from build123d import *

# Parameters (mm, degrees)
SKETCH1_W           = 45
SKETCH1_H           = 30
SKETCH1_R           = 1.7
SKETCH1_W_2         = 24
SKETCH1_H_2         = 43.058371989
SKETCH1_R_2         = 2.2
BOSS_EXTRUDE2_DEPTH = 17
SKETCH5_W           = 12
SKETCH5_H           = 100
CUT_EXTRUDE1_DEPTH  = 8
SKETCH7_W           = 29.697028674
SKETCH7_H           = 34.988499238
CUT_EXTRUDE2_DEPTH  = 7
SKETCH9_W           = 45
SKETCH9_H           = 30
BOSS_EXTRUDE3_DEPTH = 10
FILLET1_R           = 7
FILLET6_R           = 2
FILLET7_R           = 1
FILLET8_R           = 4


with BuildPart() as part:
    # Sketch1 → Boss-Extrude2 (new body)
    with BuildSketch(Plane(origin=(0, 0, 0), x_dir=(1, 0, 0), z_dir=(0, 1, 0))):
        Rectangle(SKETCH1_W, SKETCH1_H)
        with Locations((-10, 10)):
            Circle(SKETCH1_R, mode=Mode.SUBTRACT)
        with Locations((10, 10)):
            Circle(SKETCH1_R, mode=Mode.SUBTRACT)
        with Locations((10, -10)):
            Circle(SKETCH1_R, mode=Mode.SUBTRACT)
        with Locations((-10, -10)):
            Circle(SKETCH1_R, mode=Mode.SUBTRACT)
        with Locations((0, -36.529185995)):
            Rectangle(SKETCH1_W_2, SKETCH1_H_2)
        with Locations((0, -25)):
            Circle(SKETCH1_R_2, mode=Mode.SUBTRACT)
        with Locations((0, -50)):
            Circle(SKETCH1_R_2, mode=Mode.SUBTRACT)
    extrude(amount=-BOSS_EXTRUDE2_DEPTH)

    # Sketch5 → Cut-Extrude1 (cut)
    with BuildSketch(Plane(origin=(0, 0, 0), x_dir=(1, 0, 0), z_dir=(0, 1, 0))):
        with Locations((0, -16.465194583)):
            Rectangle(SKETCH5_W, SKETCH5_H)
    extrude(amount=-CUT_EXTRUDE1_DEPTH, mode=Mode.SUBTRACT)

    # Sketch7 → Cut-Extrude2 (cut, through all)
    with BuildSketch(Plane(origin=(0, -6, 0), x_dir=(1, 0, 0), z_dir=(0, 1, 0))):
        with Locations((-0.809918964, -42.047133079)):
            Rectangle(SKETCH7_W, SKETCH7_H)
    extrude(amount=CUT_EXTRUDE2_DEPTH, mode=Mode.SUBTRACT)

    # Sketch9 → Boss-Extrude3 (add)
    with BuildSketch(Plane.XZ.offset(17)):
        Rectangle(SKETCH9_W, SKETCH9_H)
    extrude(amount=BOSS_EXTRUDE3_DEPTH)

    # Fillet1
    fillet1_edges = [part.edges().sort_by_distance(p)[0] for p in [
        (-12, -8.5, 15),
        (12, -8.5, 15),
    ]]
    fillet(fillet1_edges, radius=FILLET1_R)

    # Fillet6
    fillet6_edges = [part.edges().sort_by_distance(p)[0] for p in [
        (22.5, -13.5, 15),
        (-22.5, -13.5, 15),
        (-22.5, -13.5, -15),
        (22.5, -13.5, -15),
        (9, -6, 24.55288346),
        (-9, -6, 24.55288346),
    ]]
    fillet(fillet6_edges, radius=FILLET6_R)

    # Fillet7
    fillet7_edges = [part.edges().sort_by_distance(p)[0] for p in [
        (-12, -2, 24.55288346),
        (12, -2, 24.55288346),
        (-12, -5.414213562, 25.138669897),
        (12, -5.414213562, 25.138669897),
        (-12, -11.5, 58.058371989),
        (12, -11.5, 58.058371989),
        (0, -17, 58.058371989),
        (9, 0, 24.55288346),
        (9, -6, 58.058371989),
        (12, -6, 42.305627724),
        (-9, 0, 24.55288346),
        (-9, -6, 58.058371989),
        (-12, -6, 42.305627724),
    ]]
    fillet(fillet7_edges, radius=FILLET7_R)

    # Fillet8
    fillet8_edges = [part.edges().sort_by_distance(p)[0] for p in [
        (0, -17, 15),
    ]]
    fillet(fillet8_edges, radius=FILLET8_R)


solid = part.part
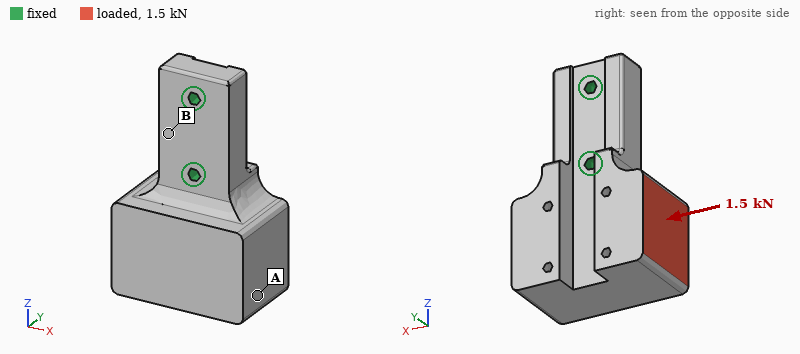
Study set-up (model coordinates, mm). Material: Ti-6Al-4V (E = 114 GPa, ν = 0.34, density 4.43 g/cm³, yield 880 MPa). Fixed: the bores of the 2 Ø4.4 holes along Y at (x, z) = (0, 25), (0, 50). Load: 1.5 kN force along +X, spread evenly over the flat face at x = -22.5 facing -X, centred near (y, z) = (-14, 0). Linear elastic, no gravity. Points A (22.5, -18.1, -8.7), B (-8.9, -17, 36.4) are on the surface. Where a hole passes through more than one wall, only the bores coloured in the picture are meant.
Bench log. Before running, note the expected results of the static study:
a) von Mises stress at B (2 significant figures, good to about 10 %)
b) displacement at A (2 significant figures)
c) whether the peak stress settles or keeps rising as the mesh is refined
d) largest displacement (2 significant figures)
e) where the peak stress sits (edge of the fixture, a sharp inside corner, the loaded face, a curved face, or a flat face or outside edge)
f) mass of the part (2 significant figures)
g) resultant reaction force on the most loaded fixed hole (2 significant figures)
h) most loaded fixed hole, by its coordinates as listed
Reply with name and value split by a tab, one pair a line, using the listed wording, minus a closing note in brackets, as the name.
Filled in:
von Mises stress at B	13 MPa
displacement at A	25 µm
whether the peak stress settles or keeps rising as the mesh is refined	keeps rising
largest displacement	28 µm
where the peak stress sits	edge of the fixture
mass of the part	200 g
resultant reaction force on the most loaded fixed hole	2.6 kN
most loaded fixed hole, by its coordinates as listed	(0, 25)
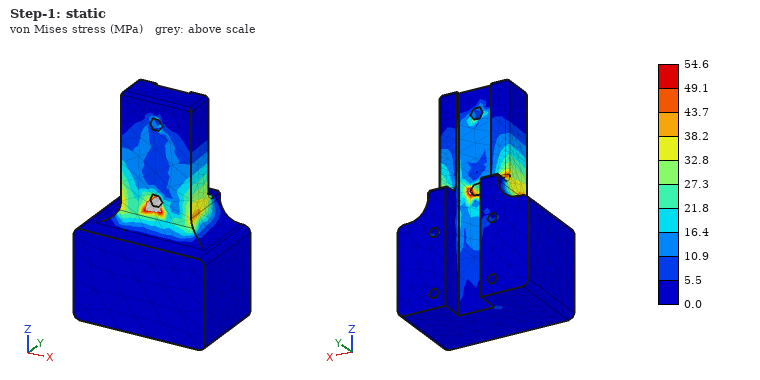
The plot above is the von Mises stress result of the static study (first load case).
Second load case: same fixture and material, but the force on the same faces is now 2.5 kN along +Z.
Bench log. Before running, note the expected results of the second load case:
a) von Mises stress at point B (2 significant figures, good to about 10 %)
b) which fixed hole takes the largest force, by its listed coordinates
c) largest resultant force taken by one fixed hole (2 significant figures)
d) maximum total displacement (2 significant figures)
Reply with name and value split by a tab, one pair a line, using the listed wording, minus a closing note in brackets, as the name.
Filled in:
von Mises stress at point B	24 MPa
which fixed hole takes the largest force, by its listed coordinates	(0, 25)
largest resultant force taken by one fixed hole	2.7 kN
maximum total displacement	45 µm
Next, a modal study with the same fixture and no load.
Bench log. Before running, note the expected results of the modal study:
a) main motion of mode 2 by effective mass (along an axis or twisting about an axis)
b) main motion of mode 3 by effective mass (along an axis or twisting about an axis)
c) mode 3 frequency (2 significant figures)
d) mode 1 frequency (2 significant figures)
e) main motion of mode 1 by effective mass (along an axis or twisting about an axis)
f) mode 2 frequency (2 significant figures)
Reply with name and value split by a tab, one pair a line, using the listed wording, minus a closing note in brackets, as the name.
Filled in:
main motion of mode 2 by effective mass	along X
main motion of mode 3 by effective mass	twisting about Z
mode 3 frequency	3900 Hz
mode 1 frequency	2500 Hz
main motion of mode 1 by effective mass	along Y
mode 2 frequency	3400 Hz
